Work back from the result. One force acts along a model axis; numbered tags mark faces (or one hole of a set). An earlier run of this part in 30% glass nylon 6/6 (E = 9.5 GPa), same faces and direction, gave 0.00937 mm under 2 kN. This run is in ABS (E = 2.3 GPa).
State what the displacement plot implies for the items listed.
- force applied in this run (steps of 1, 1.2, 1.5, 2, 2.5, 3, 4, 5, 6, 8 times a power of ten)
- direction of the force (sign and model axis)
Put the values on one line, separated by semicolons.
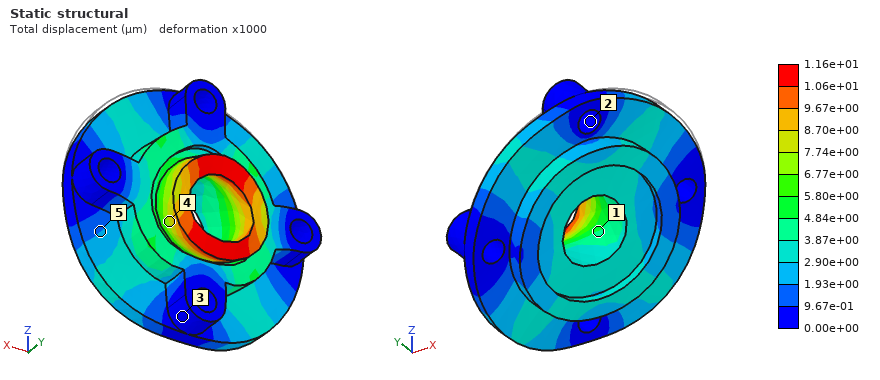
600 N; -Z
